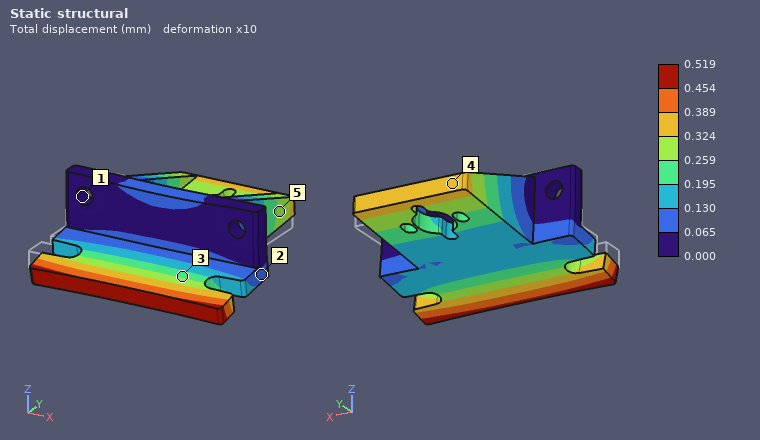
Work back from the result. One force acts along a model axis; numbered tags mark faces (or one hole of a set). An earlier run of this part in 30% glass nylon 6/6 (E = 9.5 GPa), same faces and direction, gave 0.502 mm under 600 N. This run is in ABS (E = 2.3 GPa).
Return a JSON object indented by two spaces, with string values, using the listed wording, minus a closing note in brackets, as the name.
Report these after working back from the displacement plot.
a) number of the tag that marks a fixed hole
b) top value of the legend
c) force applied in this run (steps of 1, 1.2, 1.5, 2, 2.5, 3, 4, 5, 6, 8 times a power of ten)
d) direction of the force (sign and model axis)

{
  "number of the tag that marks a fixed hole": "1",
  "top value of the legend": "0.519 mm",
  "force applied in this run": "150 N",
  "direction of the force": "-Z"
}
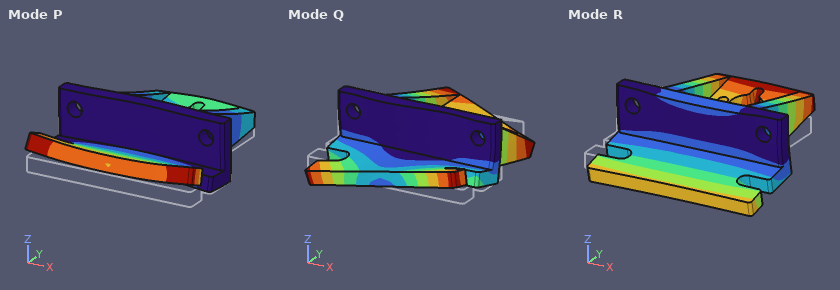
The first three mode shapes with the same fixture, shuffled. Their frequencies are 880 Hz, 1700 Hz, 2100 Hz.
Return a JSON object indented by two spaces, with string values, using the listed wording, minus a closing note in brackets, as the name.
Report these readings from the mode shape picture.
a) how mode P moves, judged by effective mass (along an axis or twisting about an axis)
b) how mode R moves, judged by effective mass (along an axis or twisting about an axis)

{
  "how mode P moves, judged by effective mass": "along Z",
  "how mode R moves, judged by effective mass": "along Y"
}
